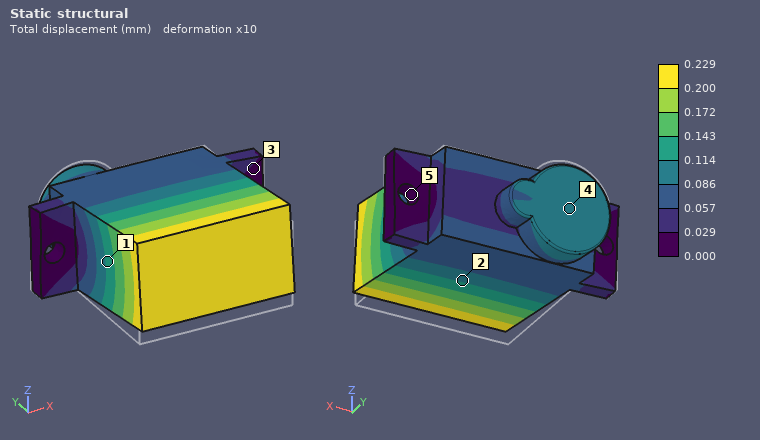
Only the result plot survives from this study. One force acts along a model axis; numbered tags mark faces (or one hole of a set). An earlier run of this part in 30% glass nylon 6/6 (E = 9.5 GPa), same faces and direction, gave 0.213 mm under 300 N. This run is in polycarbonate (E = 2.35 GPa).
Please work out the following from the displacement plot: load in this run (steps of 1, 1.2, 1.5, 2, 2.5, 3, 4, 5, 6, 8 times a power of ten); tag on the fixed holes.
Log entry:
80 N
5
